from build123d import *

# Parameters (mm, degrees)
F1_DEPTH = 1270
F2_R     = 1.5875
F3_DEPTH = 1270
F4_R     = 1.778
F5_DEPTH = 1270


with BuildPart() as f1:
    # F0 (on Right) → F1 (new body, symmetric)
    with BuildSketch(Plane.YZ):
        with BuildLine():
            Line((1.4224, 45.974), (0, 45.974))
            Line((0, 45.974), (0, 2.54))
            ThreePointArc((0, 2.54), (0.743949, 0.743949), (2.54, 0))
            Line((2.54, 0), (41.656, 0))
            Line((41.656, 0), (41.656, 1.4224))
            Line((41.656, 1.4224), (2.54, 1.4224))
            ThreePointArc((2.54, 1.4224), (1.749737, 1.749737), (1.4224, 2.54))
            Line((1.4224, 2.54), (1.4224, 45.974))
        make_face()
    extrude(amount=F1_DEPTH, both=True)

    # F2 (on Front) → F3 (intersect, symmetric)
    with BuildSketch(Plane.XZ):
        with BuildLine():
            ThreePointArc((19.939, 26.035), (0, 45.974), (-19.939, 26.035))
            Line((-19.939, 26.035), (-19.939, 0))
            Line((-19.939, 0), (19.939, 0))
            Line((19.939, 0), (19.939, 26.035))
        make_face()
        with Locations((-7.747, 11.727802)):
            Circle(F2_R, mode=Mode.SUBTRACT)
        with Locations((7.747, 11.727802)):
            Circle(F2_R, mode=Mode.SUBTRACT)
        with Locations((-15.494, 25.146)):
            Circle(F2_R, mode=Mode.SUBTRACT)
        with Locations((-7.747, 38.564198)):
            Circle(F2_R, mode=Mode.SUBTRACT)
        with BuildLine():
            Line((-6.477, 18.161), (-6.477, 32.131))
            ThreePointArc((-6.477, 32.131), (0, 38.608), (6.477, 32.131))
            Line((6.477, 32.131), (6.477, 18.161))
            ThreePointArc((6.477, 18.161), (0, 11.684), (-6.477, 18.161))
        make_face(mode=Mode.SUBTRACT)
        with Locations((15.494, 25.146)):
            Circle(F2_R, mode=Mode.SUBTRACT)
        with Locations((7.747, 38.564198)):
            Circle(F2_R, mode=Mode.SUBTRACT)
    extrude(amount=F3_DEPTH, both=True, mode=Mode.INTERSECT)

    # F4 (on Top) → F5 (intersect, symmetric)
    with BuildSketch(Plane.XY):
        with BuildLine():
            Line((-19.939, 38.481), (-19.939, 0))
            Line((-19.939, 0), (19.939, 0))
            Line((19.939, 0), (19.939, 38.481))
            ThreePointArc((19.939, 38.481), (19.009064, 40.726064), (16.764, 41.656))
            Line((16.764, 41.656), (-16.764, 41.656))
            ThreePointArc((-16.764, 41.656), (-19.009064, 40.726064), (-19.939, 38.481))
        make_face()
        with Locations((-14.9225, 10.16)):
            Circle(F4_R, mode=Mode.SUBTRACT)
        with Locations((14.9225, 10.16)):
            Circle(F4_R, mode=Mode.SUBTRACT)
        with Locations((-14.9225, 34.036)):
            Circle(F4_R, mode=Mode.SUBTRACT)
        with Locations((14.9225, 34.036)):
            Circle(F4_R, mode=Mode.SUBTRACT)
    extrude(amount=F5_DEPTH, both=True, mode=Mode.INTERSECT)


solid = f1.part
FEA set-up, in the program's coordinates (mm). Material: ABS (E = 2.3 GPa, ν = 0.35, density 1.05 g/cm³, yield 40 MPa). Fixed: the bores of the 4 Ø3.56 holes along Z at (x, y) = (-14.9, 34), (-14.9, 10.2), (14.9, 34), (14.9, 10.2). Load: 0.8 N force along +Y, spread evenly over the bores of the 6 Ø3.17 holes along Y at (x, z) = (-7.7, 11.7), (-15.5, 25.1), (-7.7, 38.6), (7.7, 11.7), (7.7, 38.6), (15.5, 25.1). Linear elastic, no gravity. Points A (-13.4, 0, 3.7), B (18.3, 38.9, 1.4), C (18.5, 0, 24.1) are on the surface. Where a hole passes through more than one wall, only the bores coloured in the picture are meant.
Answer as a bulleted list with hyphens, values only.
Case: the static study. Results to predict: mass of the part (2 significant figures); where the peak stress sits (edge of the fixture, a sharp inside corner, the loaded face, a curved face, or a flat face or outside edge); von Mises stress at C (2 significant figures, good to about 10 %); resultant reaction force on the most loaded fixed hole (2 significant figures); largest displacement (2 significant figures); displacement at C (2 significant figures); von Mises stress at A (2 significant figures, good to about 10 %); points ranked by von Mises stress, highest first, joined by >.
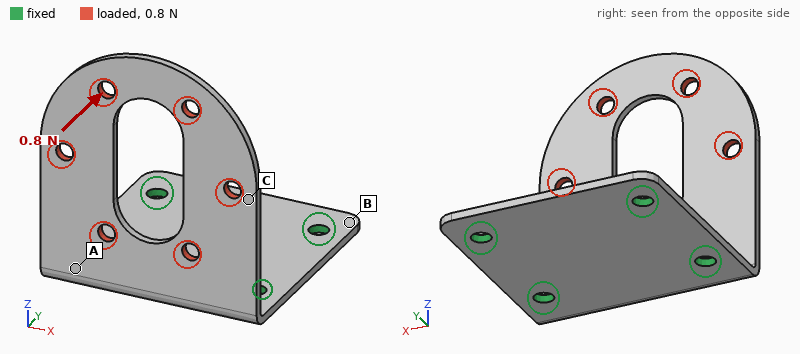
- 4.2 g
- a flat face or outside edge
- 0.56 MPa
- 0.28 N
- 0.85 mm
- 0.35 mm
- 1.2 MPa
- A > C > B
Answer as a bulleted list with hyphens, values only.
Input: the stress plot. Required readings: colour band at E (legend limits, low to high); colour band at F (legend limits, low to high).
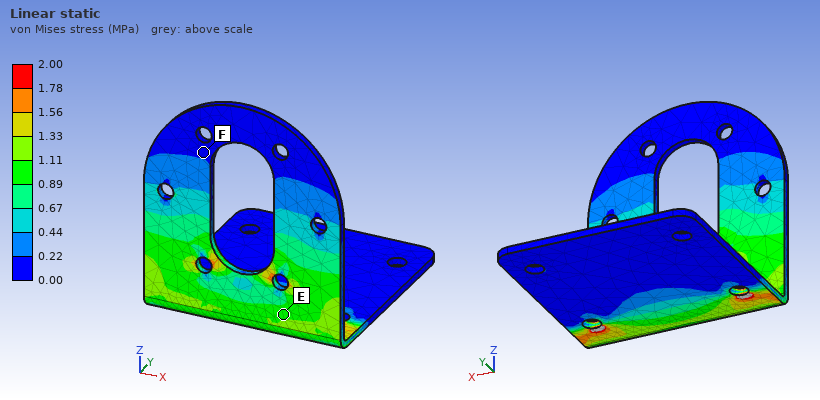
- 0.89 to 1.11 MPa
- 0.00 to 0.22 MPa
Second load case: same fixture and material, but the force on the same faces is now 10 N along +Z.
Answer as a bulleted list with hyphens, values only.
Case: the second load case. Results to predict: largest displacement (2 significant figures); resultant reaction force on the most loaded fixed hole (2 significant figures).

- 0.83 mm
- 5.3 N
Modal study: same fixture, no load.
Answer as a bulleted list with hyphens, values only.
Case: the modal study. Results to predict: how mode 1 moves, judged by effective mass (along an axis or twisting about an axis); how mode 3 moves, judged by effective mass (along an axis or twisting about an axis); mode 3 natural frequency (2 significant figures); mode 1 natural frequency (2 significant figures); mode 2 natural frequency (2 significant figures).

- along Y
- along X
- 750 Hz
- 160 Hz
- 440 Hz
